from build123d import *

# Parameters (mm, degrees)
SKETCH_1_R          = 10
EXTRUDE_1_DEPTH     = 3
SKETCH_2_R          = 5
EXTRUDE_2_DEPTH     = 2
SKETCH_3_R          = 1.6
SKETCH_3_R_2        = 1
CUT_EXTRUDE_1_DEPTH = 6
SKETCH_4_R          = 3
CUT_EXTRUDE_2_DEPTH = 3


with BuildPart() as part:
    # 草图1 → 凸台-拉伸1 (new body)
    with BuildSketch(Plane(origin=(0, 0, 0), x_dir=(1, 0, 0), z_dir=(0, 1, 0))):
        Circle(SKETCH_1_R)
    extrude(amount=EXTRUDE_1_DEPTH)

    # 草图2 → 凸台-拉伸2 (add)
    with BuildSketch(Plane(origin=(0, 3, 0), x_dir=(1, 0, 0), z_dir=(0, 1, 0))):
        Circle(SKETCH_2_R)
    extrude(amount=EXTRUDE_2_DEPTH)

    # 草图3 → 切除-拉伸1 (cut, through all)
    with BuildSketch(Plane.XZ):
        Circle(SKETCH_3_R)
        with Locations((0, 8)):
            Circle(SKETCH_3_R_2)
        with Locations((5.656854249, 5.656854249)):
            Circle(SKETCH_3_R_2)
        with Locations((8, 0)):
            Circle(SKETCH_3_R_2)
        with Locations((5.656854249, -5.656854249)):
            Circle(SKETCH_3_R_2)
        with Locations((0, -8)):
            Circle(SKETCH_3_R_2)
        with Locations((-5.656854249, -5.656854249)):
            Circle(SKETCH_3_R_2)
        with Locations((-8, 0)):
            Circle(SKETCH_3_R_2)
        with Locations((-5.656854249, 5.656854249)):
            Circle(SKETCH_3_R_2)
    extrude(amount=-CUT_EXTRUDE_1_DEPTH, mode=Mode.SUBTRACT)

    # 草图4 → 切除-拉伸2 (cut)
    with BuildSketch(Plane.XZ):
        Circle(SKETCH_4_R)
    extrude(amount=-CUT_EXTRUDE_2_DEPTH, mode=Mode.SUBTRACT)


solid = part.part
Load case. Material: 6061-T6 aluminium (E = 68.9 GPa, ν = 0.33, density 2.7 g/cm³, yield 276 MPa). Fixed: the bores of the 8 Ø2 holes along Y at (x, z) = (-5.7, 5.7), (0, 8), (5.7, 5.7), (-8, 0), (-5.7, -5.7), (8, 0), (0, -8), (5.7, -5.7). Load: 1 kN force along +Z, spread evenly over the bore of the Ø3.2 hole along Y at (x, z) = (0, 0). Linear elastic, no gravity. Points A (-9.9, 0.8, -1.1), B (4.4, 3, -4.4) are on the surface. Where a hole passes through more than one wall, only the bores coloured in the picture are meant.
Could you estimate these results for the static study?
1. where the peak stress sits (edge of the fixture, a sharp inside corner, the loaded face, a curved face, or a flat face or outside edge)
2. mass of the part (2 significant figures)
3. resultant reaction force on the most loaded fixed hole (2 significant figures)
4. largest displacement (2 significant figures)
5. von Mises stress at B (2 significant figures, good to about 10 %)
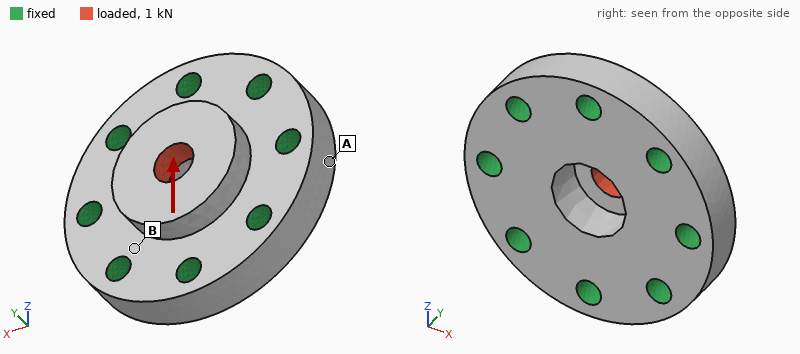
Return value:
the loaded face
2.5 g
220 N
5.0 µm
23 MPa
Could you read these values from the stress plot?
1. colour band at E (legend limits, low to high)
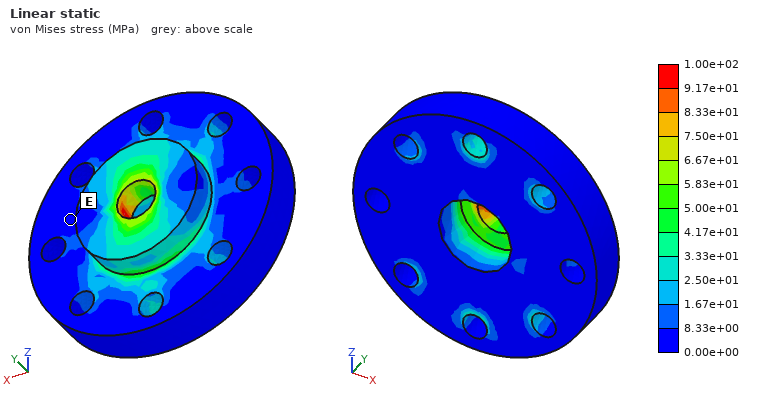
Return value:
0.00e+00 to 8.33e+00 MPa
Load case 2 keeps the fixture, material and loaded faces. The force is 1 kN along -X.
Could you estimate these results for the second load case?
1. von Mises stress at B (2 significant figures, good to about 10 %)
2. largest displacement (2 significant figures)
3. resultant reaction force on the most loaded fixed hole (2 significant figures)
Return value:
23 MPa
5.0 µm
220 N
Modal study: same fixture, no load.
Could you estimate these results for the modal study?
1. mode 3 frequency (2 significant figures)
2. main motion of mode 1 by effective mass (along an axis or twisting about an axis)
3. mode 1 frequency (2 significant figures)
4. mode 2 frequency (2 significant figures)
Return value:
140 kHz
along Y
100 kHz
140 kHz
